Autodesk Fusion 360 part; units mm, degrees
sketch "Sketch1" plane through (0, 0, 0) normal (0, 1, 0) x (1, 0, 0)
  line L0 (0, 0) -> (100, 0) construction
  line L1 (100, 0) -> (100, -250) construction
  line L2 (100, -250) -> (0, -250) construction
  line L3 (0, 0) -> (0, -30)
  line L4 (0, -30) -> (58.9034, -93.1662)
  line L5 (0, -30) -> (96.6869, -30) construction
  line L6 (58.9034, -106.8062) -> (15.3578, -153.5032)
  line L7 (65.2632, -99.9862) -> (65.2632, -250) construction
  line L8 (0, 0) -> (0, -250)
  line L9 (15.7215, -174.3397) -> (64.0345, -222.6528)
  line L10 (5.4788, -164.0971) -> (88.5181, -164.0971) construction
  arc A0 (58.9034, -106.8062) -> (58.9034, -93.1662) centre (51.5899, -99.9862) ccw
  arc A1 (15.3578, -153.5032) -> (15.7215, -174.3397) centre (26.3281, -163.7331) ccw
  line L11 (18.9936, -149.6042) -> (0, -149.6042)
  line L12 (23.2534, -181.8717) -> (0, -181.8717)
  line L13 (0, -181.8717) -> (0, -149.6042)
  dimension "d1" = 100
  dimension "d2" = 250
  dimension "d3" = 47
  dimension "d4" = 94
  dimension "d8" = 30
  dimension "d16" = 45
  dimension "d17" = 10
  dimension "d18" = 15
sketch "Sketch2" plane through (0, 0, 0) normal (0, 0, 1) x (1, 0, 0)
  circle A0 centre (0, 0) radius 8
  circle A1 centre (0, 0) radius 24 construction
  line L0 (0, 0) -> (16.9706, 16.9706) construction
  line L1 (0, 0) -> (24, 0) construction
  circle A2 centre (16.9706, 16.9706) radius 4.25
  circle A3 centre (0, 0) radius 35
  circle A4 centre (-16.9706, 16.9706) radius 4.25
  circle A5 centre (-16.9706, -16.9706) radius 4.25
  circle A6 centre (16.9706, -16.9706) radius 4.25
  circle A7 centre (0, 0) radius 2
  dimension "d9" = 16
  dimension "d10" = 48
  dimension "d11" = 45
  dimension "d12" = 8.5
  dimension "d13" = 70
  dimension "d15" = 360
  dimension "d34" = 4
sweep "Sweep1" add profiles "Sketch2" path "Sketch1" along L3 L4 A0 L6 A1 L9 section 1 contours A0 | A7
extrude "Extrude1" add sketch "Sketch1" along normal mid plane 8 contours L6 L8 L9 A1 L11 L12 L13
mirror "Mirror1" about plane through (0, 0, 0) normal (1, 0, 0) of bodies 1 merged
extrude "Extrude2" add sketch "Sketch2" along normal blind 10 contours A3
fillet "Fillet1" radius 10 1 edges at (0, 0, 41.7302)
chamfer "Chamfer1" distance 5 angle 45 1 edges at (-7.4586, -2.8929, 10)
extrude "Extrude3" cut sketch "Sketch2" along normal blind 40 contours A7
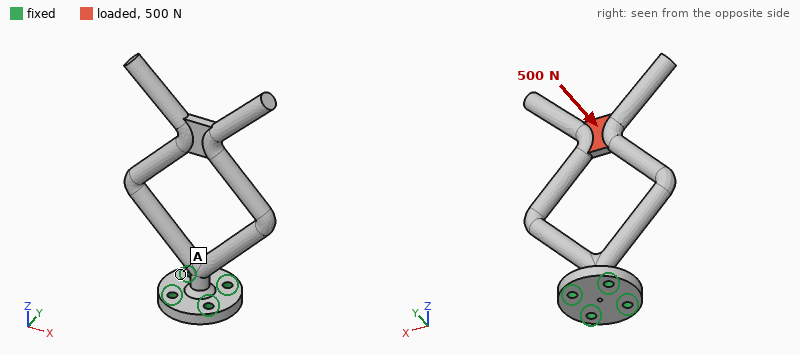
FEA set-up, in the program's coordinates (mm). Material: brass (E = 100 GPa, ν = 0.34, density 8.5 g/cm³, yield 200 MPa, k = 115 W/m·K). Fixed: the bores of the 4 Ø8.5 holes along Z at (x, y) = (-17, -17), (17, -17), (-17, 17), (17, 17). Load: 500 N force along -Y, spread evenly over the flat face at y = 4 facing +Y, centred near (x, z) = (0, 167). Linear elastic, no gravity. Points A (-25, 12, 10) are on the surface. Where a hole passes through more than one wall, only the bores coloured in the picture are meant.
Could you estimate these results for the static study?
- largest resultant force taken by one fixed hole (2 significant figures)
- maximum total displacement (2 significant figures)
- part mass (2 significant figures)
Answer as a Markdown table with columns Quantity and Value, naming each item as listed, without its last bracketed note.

| Quantity | Value |
|---|---|
| largest resultant force taken by one fixed hole | 1.4 kN |
| maximum total displacement | 2.7 mm |
| part mass | 1.2 kg |
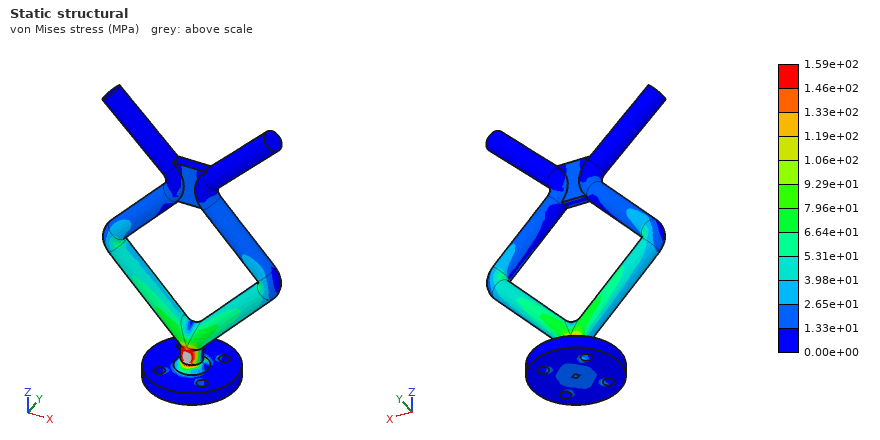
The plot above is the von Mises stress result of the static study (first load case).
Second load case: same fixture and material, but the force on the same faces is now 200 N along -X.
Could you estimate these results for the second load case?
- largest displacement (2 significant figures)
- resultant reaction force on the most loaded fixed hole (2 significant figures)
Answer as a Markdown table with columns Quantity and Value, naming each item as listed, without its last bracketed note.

| Quantity | Value |
|---|---|
| largest displacement | 0.60 mm |
| resultant reaction force on the most loaded fixed hole | 560 N |
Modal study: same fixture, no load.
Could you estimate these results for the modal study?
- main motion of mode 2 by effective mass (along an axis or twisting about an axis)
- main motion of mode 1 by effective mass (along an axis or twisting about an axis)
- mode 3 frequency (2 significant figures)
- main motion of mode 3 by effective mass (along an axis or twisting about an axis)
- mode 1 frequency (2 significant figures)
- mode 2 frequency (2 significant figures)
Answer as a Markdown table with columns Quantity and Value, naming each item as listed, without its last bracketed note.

| Quantity | Value |
|---|---|
| main motion of mode 2 by effective mass | along X |
| main motion of mode 1 by effective mass | along Y |
| mode 3 frequency | 320 Hz |
| main motion of mode 3 by effective mass | twisting about Z |
| mode 1 frequency | 110 Hz |
| mode 2 frequency | 140 Hz |
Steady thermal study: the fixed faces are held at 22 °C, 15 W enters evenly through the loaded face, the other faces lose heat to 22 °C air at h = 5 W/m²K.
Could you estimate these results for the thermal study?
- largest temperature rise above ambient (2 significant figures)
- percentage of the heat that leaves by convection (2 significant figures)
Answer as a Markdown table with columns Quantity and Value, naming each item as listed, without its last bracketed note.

| Quantity | Value |
|---|---|
| largest temperature rise above ambient | 55 K |
| percentage of the heat that leaves by convection | 33 % |
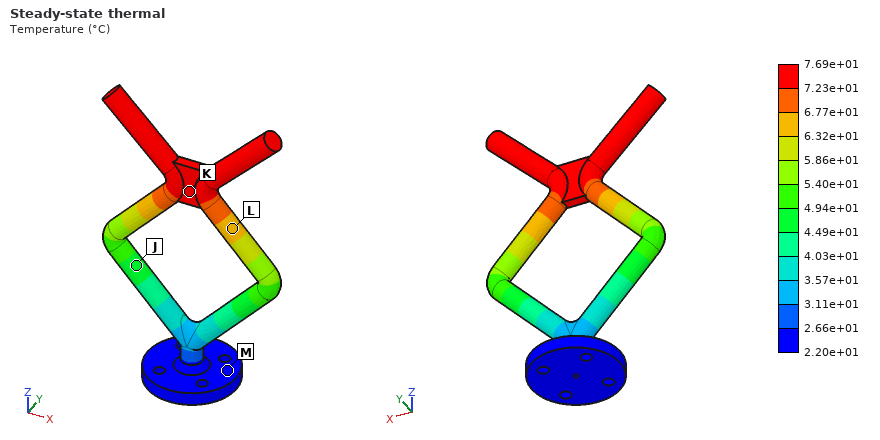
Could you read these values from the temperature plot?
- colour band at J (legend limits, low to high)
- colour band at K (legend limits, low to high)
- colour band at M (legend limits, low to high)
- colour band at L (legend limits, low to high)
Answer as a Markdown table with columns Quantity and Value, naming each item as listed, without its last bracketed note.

| Quantity | Value |
|---|---|
| colour band at J | 4.49e+01 to 4.94e+01 °C |
| colour band at K | 7.23e+01 to 7.69e+01 °C |
| colour band at M | 2.20e+01 to 2.66e+01 °C |
| colour band at L | 6.32e+01 to 6.77e+01 °C |
